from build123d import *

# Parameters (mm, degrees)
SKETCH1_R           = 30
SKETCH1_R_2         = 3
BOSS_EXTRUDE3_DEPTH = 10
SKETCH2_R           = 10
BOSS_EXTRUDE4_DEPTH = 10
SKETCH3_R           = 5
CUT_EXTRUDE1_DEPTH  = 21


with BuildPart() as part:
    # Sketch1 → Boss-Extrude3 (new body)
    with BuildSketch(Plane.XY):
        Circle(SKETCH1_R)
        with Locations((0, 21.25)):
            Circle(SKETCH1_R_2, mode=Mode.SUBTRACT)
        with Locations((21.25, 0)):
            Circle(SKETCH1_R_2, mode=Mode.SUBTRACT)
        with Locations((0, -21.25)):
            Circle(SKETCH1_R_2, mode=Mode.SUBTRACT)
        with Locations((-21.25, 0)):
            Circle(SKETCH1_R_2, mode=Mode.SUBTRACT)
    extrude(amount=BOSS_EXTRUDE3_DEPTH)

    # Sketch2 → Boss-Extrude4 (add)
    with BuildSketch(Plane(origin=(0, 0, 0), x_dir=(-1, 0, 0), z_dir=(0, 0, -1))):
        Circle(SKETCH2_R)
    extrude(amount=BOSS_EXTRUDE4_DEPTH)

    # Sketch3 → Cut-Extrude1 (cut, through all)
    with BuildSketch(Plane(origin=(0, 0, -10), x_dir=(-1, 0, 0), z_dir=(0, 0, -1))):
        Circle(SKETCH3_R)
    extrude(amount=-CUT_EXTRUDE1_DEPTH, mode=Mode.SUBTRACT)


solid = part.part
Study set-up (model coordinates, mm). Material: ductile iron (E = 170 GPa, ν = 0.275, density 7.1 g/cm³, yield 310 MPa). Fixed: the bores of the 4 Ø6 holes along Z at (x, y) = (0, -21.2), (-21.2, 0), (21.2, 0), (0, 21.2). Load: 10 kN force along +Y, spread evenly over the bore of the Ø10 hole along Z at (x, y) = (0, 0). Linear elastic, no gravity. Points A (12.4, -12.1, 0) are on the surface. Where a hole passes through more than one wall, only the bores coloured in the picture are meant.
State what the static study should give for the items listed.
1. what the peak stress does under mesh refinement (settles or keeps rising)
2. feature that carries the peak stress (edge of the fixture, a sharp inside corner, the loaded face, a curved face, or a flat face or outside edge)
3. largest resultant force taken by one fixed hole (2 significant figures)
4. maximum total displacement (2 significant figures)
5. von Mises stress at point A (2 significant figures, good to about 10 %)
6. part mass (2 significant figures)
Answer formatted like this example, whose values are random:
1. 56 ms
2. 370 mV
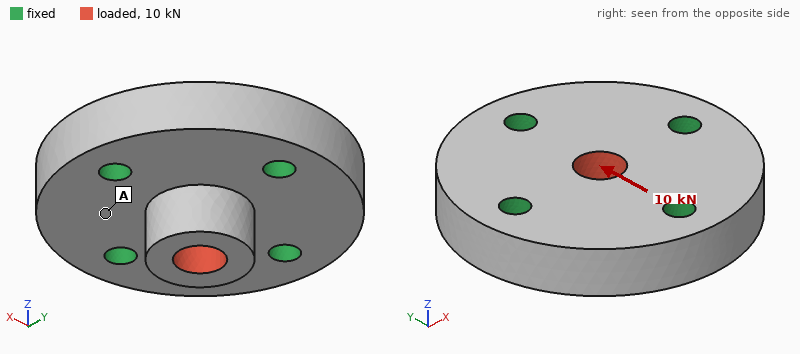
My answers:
1. keeps rising
2. edge of the fixture
3. 3.5 kN
4. 8.5 µm
5. 9.0 MPa
6. 200 g
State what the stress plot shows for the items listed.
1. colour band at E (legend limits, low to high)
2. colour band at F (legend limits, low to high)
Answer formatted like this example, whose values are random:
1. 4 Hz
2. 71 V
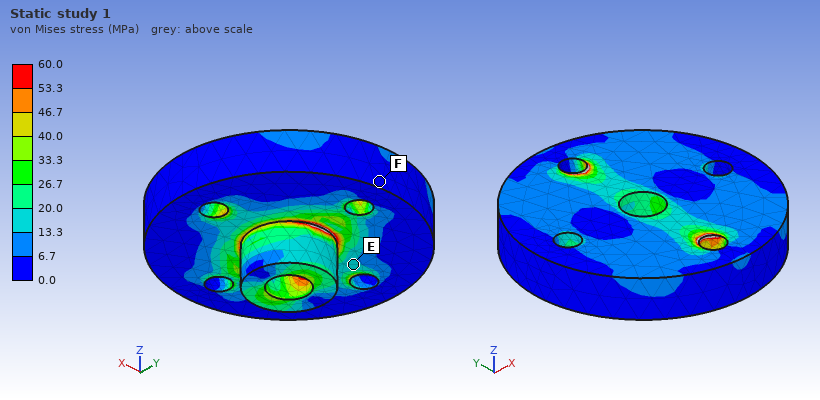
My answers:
1. 13.3 to 20.0 MPa
2. 0.0 to 6.7 MPa
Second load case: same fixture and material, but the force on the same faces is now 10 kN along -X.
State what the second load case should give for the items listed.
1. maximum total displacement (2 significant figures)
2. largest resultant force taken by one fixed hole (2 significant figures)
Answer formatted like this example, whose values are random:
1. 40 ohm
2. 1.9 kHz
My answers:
1. 8.4 µm
2. 3.5 kN
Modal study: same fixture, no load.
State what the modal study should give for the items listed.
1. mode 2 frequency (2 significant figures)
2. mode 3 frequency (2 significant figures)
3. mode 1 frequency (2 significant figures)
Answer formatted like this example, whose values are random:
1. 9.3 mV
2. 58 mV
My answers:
1. 28 kHz
2. 28 kHz
3. 27 kHz
